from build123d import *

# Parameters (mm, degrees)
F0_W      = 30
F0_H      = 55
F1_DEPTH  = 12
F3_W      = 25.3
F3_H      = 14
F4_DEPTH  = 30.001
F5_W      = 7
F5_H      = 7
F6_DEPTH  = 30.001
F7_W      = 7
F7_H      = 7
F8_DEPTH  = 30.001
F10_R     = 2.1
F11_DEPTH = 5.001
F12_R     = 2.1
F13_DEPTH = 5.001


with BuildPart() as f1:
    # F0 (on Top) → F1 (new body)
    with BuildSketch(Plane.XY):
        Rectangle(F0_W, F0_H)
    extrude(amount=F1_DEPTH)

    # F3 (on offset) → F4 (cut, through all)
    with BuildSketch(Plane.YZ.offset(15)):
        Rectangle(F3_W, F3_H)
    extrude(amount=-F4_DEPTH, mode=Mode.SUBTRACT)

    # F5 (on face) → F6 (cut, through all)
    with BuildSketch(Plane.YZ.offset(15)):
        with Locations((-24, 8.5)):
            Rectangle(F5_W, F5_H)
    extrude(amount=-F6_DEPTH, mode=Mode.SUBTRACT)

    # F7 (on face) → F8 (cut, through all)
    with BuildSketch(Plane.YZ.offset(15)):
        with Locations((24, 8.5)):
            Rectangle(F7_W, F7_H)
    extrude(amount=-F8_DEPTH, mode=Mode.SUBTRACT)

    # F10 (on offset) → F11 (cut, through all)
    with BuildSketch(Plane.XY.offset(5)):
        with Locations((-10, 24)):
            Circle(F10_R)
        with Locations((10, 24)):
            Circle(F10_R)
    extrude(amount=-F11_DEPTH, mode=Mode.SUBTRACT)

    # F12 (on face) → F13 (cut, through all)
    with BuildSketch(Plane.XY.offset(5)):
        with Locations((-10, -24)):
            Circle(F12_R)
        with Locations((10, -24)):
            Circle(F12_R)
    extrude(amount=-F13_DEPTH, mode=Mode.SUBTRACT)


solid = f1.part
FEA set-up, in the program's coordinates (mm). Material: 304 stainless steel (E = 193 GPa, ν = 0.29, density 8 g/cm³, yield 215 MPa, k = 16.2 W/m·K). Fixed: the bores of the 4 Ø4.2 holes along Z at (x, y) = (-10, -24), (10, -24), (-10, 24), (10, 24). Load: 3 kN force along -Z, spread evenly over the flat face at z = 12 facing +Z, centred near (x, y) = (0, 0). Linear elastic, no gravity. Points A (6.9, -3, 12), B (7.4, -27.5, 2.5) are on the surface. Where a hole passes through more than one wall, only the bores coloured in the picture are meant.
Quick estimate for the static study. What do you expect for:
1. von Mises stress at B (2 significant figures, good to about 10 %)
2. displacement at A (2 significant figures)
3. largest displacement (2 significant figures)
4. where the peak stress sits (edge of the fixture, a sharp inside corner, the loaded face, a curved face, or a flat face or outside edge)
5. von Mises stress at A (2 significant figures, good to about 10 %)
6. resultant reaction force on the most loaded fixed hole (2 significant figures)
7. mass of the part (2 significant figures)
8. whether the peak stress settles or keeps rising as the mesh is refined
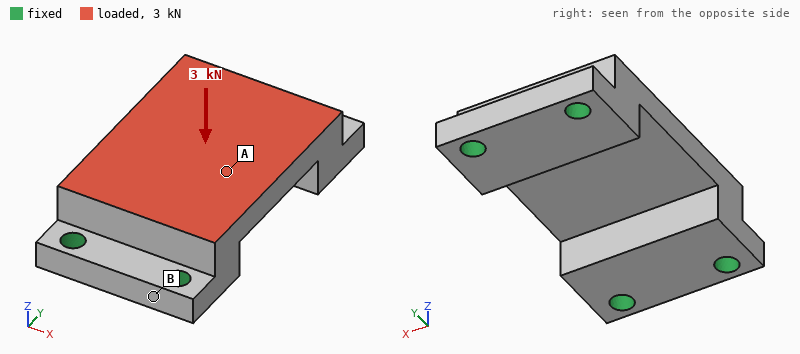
11 MPa
6.2 µm
6.9 µm
edge of the fixture
31 MPa
1.1 kN
90 g
keeps rising
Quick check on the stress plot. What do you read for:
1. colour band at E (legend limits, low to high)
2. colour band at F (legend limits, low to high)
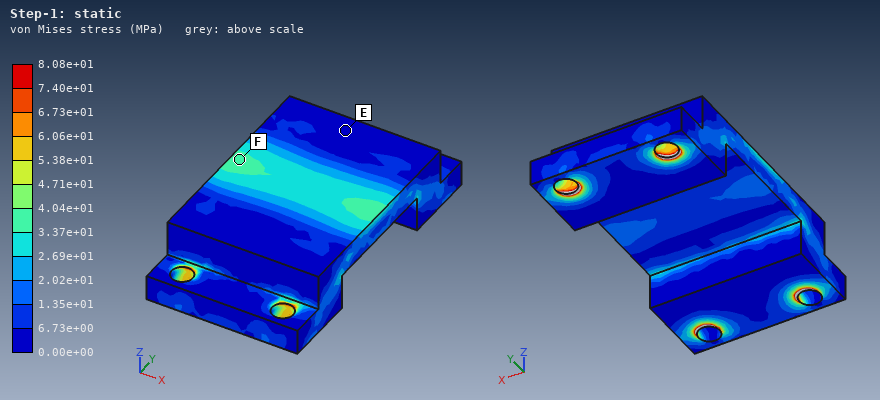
0.00e+00 to 6.73e+00 MPa
3.37e+01 to 4.04e+01 MPa
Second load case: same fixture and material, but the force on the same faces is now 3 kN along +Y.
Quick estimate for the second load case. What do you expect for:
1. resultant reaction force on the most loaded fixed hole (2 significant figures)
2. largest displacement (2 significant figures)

810 N
3.7 µm
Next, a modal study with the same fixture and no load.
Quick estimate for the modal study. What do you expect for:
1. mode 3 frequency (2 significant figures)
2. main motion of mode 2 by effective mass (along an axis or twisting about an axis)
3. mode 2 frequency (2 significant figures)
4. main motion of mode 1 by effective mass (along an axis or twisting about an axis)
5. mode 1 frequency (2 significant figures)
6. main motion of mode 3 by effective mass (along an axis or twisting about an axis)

20 kHz
along Y
18 kHz
along Z
17 kHz
along X
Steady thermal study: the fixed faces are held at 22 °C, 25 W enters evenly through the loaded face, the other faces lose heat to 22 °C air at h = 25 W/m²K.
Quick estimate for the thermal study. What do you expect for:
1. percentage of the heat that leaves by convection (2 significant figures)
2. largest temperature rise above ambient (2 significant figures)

12 %
70 K
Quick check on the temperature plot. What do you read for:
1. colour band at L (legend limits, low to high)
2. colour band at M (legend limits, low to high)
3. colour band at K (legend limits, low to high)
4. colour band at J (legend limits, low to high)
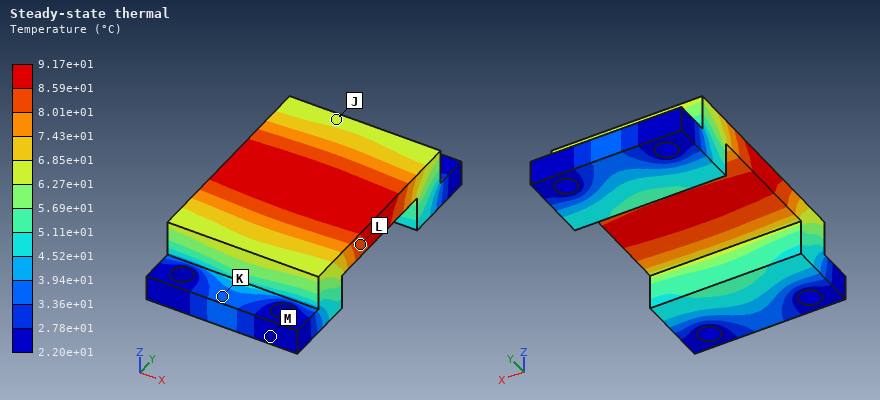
8.01e+01 to 8.59e+01 °C
2.20e+01 to 2.78e+01 °C
3.36e+01 to 3.94e+01 °C
6.27e+01 to 6.85e+01 °C
